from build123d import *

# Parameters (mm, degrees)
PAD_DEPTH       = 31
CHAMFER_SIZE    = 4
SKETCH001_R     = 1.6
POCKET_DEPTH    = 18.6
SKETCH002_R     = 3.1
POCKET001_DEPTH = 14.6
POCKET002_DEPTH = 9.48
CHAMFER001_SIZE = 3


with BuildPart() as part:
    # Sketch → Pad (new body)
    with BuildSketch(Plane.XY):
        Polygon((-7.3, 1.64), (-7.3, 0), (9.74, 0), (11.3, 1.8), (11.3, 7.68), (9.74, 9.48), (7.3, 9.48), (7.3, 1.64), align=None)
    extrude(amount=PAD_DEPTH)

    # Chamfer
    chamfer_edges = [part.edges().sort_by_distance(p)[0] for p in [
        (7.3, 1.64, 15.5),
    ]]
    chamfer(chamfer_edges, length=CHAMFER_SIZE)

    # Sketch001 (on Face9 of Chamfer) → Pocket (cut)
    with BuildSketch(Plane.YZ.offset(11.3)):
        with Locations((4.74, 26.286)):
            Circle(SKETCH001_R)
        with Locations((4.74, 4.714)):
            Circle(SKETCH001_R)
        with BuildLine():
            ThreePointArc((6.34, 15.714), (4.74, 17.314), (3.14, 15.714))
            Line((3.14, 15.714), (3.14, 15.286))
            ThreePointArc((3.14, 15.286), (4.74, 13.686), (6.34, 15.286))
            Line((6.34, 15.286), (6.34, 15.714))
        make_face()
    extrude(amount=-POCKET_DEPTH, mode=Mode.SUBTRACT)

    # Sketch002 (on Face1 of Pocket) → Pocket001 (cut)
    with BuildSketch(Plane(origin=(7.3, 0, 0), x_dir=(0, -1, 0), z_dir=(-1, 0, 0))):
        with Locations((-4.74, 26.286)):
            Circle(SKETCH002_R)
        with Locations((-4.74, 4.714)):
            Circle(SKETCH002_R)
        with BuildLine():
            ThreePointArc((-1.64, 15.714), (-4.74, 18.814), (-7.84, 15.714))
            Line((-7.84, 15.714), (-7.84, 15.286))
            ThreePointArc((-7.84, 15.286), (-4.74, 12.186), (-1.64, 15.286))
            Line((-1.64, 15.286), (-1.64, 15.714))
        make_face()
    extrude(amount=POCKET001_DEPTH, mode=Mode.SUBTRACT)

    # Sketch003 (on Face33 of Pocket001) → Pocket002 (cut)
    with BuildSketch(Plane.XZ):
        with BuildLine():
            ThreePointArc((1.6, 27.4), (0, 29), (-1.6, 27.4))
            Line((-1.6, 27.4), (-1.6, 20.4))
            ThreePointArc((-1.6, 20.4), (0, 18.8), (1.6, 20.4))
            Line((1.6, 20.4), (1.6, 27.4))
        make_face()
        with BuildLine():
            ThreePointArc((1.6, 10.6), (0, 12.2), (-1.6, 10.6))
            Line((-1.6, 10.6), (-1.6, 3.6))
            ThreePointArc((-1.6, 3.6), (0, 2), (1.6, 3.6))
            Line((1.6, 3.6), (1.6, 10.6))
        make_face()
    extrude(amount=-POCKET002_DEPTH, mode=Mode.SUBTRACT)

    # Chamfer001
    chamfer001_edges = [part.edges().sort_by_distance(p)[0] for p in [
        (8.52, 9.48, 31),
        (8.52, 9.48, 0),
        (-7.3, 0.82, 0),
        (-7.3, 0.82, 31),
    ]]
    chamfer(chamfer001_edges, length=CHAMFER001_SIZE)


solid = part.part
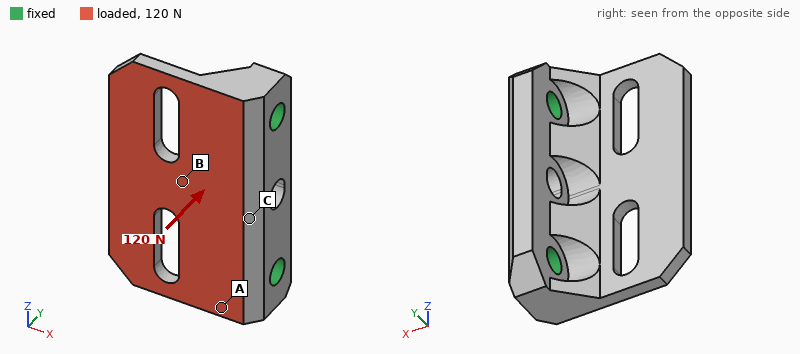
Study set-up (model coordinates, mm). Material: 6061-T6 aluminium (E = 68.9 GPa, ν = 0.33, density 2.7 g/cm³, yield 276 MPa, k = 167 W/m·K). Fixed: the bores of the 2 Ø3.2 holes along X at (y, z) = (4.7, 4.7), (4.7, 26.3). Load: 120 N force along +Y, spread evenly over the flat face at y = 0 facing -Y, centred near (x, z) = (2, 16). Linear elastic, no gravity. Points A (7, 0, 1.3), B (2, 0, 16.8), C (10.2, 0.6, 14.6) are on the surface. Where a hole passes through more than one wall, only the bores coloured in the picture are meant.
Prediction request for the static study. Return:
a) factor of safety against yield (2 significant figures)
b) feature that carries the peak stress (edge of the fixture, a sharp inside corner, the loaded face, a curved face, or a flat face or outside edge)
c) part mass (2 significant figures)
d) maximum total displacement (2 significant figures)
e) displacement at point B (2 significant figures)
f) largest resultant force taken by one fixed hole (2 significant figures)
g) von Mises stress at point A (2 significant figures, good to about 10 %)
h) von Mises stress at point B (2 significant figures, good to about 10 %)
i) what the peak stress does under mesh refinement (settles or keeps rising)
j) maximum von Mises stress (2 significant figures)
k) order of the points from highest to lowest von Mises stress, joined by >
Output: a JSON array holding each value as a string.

["4.2", "the loaded face", "4.6 g", "54 µm", "8.8 µm", "60 N", "11 MPa", "42 MPa", "settles", "66 MPa", "B > A > C"]
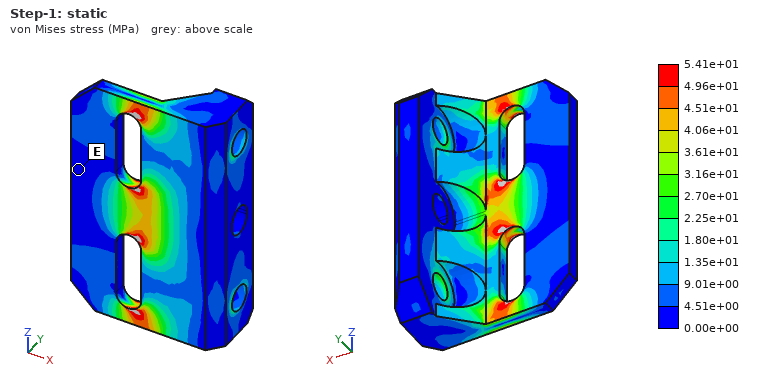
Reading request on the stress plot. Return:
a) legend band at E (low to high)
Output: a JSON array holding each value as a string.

["0.00e+00 to 4.51e+00 MPa"]
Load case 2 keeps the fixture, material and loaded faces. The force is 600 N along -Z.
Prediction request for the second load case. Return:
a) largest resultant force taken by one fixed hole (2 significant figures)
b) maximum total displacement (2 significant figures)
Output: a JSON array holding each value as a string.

["370 N", "13 µm"]
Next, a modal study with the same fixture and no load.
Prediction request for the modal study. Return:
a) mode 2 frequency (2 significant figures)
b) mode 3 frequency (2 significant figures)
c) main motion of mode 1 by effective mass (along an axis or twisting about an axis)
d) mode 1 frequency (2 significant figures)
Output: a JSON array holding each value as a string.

["10 kHz", "19 kHz", "along Y", "6500 Hz"]
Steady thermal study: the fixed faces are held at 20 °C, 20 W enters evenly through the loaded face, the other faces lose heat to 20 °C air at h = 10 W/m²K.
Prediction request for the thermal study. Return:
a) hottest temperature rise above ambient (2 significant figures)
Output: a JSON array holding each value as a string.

["29 K"]
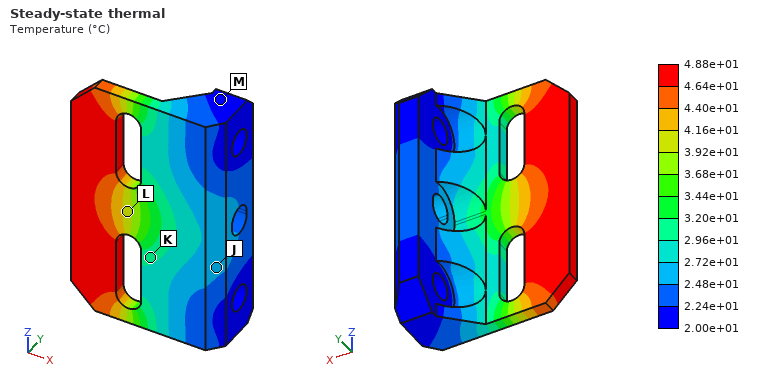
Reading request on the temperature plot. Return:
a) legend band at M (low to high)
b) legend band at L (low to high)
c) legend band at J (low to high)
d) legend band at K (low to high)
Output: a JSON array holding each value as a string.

["2.00e+01 to 2.24e+01 °C", "3.92e+01 to 4.16e+01 °C", "2.48e+01 to 2.72e+01 °C", "2.96e+01 to 3.20e+01 °C"]
